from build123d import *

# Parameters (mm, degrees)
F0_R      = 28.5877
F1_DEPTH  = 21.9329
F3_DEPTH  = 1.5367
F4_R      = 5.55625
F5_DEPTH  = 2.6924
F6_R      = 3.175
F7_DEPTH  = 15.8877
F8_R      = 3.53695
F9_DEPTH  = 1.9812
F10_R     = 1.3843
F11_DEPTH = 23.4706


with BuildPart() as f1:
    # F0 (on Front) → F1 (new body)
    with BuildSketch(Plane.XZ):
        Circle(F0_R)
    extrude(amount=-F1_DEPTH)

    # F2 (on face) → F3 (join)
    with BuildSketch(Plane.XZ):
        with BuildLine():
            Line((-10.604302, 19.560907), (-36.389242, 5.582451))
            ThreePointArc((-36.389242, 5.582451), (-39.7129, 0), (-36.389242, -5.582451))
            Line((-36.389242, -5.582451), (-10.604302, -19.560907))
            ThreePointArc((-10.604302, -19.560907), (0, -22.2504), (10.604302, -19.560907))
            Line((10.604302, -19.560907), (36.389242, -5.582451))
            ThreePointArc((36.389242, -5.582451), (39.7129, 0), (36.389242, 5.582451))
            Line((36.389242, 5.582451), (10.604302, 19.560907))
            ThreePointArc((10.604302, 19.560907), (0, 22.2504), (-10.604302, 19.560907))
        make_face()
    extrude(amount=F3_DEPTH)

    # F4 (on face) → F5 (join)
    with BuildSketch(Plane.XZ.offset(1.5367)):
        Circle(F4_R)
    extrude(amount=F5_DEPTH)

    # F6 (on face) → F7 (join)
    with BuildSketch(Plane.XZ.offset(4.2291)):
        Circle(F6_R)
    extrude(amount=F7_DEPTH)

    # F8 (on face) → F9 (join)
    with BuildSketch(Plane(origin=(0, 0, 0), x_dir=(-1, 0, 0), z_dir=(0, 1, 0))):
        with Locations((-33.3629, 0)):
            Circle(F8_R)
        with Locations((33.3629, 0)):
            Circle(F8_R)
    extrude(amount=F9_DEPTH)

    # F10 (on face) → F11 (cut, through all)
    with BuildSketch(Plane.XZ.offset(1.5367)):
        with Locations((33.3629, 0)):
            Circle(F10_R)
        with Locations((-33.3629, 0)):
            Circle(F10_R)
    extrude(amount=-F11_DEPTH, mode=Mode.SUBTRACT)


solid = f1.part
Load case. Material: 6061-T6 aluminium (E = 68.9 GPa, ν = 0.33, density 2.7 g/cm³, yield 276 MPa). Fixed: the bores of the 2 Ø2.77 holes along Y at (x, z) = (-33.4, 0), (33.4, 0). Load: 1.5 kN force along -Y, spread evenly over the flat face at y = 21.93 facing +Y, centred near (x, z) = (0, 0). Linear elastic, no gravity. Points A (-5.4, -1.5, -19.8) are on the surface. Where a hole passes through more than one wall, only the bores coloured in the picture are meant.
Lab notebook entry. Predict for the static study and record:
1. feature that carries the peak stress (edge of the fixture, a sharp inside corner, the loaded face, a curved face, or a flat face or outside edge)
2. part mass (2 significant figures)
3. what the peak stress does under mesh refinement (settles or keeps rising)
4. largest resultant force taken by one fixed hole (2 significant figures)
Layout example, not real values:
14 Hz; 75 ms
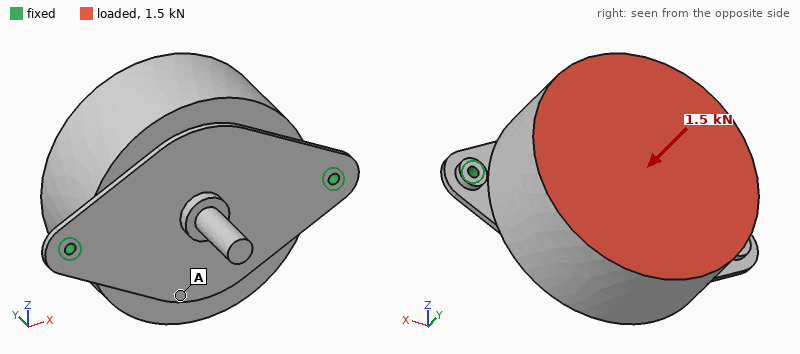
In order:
edge of the fixture; 160 g; keeps rising; 780 N
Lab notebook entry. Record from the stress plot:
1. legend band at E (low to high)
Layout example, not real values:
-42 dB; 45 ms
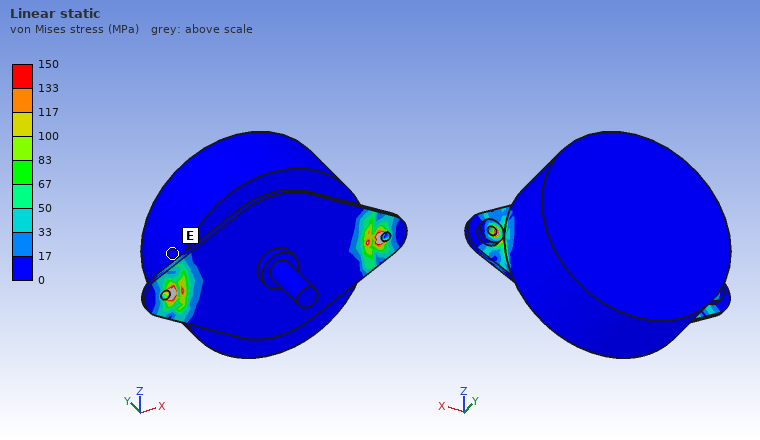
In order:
0 to 17 MPa
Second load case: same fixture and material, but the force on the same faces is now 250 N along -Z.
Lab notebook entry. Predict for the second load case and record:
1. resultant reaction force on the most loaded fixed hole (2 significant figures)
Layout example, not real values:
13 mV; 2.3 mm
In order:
130 N
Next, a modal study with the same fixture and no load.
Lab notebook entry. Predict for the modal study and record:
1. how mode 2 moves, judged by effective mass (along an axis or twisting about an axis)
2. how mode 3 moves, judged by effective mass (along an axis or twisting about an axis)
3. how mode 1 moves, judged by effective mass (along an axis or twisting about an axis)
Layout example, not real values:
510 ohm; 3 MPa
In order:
along Y; along X; along Z
